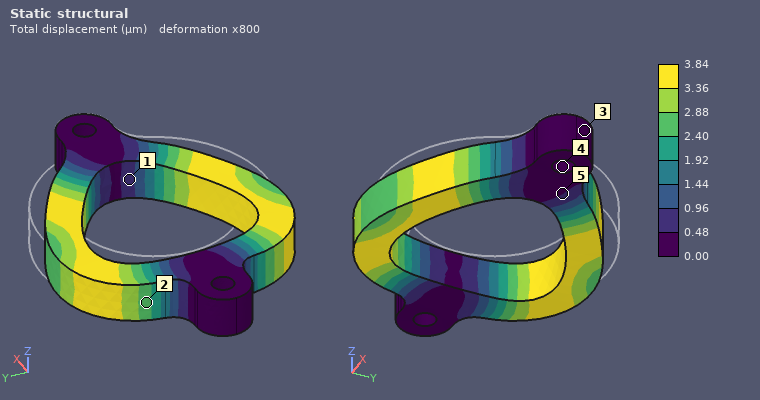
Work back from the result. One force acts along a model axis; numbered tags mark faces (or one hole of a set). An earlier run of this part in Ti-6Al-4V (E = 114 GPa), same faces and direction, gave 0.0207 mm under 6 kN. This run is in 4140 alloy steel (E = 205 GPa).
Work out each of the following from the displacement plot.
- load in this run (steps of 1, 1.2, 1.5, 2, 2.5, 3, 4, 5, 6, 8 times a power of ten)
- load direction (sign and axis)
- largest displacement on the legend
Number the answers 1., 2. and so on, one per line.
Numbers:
1. 2 kN
2. -X
3. 3.84 µm
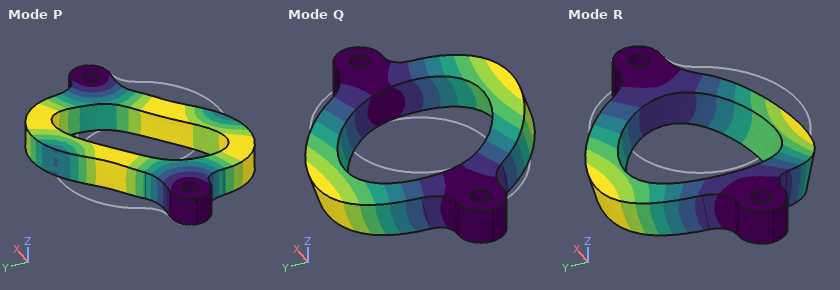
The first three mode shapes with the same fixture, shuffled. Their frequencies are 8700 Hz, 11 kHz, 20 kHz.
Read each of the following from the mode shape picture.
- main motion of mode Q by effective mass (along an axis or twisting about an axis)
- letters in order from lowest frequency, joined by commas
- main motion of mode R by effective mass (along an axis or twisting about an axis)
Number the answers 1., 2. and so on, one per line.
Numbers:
1. twisting about X
2. Q, R, P
3. along Z
